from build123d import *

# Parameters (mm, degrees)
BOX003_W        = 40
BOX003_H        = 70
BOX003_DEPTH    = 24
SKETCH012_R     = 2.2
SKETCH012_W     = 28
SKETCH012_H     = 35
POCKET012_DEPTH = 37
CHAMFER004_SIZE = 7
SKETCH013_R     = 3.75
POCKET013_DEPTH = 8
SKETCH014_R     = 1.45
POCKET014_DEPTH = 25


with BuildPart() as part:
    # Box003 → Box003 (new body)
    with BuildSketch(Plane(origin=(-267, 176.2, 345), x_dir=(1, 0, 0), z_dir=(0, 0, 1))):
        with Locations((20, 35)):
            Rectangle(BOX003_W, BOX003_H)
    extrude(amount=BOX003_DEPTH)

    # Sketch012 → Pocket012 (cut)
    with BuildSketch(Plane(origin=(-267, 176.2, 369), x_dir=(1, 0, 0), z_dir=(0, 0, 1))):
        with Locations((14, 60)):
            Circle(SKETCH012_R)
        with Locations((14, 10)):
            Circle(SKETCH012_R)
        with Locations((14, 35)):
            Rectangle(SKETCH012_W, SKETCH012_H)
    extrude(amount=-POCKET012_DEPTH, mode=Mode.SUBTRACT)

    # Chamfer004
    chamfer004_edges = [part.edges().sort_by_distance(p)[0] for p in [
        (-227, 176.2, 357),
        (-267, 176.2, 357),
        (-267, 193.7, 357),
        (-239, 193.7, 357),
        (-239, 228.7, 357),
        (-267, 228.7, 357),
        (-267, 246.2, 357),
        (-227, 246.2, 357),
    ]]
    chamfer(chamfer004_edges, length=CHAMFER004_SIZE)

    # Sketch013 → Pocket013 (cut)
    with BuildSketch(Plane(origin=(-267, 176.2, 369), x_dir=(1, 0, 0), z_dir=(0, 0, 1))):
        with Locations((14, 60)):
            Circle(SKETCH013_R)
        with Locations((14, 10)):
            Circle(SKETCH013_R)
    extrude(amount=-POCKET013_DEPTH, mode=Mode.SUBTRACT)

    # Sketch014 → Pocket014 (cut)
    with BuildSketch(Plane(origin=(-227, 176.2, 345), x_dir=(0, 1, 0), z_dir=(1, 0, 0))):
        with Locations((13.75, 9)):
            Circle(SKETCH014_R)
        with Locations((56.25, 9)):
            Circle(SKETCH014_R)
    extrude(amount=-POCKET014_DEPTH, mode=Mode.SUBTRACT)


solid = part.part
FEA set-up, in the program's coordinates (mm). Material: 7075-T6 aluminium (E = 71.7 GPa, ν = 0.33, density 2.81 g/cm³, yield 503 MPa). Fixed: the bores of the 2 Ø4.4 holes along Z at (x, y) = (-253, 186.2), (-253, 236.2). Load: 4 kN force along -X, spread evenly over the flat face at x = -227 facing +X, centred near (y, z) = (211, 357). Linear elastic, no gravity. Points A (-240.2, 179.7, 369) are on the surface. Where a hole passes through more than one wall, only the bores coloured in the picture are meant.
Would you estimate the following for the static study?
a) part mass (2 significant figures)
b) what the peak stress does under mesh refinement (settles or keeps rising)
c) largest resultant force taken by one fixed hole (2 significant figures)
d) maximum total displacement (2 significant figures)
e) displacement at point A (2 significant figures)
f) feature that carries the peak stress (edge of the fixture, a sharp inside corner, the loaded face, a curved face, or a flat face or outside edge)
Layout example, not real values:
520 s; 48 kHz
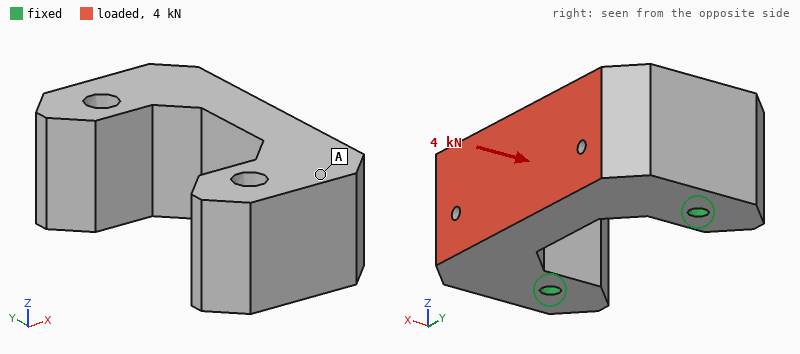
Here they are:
110 g; keeps rising; 2.2 kN; 8.7 µm; 2.7 µm; edge of the fixture
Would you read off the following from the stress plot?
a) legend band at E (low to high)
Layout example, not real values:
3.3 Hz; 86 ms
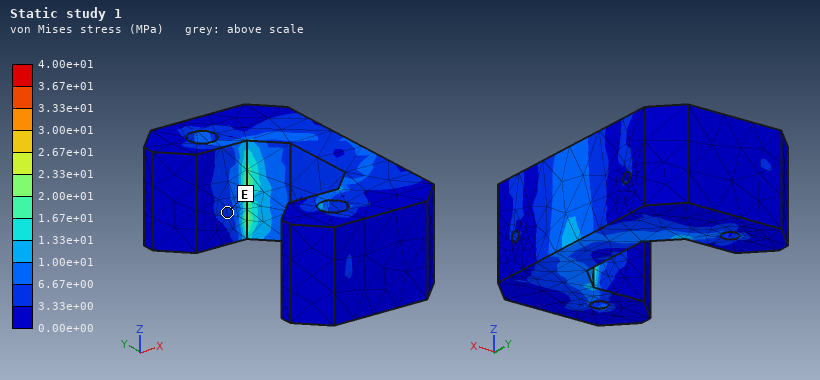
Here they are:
3.33e+00 to 6.67e+00 MPa
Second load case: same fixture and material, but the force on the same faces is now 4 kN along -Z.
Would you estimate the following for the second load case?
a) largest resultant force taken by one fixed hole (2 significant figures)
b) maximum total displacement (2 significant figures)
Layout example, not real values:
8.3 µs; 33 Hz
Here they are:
2.0 kN; 38 µm
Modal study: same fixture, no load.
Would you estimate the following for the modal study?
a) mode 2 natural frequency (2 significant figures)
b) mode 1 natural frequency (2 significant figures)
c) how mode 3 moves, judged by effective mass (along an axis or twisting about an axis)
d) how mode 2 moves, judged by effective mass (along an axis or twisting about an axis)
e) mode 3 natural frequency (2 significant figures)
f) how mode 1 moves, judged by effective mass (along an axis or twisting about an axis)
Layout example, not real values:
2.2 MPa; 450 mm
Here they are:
12 kHz; 9400 Hz; twisting about X; along Y; 15 kHz; along Z
